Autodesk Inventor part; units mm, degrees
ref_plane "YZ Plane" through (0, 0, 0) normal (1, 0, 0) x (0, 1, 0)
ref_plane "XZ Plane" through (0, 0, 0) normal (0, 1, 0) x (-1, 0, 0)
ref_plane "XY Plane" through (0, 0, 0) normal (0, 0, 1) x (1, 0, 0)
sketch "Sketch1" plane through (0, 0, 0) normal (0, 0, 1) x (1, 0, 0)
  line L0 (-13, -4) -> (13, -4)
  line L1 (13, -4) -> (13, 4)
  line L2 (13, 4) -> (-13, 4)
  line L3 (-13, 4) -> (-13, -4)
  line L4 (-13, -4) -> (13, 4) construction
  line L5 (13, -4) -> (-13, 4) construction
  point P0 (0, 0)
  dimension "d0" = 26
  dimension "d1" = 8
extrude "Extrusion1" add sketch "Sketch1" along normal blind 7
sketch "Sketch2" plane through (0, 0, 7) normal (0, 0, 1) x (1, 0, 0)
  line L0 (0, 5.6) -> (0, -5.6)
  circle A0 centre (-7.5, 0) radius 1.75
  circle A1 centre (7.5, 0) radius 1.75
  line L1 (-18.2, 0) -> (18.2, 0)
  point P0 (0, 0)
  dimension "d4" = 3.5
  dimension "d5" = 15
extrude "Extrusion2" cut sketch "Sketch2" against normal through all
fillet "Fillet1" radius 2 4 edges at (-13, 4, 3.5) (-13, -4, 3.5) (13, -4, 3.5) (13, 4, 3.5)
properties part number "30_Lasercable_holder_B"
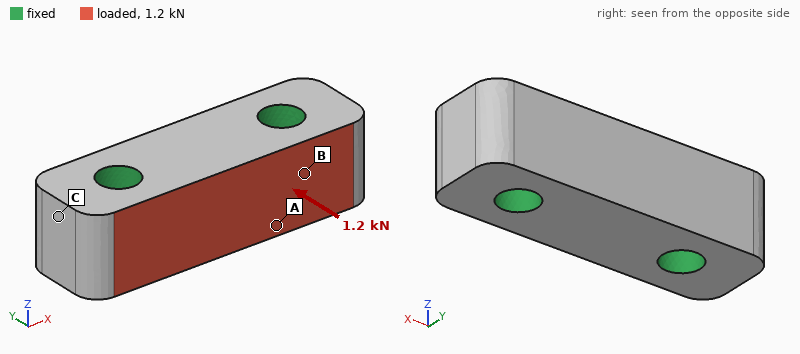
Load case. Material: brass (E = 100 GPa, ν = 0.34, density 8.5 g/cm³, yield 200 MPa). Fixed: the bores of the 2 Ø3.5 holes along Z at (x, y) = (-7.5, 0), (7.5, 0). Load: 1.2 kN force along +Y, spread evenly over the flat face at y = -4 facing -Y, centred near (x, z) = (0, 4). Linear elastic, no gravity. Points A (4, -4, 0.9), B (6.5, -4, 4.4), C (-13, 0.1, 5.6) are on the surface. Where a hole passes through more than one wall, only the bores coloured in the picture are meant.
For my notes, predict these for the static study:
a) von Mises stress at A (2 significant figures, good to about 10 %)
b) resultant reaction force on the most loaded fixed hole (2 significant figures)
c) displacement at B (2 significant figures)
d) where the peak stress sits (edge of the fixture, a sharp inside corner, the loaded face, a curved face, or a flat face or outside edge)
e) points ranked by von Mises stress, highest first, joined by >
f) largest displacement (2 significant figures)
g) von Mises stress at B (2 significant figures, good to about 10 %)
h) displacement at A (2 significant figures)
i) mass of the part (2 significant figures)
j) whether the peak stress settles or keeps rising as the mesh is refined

6.9 MPa
600 N
0.34 µm
edge of the fixture
B > A > C
1.1 µm
12 MPa
0.74 µm
11 g
keeps rising
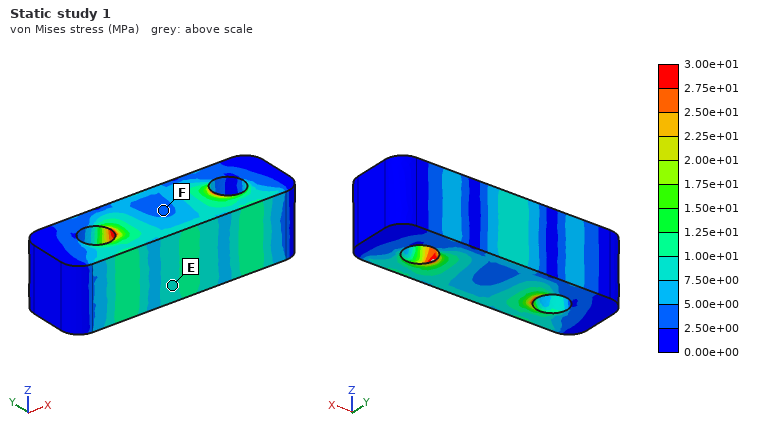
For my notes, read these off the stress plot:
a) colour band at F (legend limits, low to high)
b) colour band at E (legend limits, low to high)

2.50e+00 to 5.00e+00 MPa
7.50e+00 to 1.00e+01 MPa
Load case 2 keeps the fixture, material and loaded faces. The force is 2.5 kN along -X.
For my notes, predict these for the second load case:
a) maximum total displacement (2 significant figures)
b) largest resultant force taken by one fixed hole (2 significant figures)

1.8 µm
1.3 kN
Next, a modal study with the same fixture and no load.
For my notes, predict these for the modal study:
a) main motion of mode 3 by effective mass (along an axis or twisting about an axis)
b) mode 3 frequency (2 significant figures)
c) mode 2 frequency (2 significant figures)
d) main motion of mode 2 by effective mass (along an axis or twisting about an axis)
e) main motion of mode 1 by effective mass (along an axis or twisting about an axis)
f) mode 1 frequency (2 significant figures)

twisting about X
72 kHz
65 kHz
along Z
along Y
61 kHz
